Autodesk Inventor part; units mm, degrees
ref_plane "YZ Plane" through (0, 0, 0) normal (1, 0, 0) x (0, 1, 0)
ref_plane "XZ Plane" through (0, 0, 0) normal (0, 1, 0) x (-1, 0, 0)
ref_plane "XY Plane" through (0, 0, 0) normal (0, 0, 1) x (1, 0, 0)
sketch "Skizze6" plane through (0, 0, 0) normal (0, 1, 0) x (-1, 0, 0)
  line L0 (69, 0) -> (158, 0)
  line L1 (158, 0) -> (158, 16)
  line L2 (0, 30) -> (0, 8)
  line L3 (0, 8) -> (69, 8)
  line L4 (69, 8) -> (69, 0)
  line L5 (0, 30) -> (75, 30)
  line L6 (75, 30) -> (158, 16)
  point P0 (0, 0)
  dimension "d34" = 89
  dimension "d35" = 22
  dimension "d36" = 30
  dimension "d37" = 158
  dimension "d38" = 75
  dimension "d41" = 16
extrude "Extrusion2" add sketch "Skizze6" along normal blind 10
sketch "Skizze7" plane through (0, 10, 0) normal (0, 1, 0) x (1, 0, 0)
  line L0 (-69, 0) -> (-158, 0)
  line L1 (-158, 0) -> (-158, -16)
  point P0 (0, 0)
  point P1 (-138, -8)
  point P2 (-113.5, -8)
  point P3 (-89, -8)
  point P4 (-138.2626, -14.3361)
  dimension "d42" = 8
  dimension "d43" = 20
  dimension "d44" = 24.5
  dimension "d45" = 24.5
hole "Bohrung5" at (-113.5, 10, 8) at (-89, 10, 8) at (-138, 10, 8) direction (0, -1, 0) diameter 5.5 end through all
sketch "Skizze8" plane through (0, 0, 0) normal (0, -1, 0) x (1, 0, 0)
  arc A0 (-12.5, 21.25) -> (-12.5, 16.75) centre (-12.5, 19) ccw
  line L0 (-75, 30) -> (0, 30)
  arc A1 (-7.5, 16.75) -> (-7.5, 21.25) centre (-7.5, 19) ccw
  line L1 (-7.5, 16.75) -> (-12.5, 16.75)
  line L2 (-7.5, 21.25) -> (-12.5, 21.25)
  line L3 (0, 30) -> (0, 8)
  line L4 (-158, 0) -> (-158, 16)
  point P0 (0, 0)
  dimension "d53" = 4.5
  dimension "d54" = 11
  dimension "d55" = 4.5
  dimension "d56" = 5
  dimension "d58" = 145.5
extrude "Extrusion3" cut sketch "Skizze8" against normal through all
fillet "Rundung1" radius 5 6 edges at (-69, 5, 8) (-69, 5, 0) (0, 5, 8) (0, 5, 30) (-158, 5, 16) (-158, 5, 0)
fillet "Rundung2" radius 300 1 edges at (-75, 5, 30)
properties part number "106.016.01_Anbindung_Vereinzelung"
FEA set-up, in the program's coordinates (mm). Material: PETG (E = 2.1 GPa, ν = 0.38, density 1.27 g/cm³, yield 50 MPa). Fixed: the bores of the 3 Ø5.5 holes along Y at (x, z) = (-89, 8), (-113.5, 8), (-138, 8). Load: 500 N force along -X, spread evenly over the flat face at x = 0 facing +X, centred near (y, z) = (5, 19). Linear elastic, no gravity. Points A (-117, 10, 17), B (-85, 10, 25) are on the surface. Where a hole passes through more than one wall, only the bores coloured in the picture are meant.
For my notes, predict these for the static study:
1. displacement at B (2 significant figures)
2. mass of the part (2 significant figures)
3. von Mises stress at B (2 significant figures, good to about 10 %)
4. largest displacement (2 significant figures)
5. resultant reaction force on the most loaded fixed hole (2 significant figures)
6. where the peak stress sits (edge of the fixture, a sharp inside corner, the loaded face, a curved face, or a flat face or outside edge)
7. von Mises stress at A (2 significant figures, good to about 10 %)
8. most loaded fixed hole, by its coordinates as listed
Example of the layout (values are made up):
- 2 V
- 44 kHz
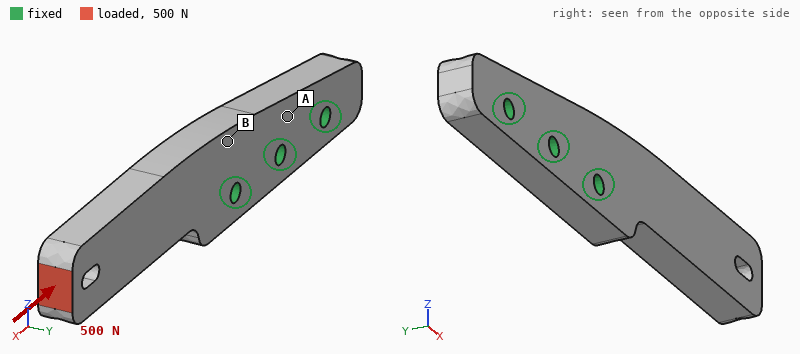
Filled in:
- 0.045 mm
- 44 g
- 3.0 MPa
- 0.30 mm
- 340 N
- a curved face
- 0.82 MPa
- (-89, 8)
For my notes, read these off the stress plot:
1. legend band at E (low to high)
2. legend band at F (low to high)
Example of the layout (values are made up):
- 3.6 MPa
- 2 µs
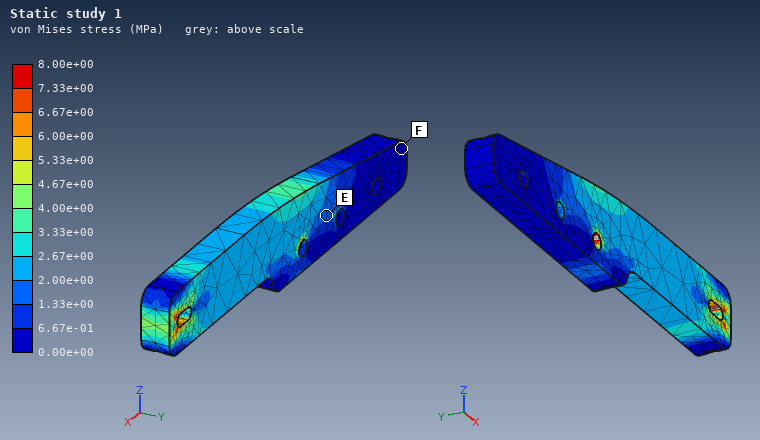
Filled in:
- 1.33e+00 to 2.00e+00 MPa
- 0.00e+00 to 6.67e-01 MPa
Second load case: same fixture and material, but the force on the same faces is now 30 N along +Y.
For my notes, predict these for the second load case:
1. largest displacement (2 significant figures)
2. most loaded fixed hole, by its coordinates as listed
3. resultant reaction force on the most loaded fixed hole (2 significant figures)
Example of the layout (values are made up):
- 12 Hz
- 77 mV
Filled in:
- 1.8 mm
- (-89, 8)
- 68 N
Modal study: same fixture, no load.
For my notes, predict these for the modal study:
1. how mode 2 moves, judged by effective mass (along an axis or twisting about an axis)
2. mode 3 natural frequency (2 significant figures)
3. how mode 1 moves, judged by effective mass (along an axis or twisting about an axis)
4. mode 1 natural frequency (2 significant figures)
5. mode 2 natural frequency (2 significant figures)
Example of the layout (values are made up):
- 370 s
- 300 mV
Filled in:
- along Z
- 1400 Hz
- along Y
- 280 Hz
- 570 Hz
